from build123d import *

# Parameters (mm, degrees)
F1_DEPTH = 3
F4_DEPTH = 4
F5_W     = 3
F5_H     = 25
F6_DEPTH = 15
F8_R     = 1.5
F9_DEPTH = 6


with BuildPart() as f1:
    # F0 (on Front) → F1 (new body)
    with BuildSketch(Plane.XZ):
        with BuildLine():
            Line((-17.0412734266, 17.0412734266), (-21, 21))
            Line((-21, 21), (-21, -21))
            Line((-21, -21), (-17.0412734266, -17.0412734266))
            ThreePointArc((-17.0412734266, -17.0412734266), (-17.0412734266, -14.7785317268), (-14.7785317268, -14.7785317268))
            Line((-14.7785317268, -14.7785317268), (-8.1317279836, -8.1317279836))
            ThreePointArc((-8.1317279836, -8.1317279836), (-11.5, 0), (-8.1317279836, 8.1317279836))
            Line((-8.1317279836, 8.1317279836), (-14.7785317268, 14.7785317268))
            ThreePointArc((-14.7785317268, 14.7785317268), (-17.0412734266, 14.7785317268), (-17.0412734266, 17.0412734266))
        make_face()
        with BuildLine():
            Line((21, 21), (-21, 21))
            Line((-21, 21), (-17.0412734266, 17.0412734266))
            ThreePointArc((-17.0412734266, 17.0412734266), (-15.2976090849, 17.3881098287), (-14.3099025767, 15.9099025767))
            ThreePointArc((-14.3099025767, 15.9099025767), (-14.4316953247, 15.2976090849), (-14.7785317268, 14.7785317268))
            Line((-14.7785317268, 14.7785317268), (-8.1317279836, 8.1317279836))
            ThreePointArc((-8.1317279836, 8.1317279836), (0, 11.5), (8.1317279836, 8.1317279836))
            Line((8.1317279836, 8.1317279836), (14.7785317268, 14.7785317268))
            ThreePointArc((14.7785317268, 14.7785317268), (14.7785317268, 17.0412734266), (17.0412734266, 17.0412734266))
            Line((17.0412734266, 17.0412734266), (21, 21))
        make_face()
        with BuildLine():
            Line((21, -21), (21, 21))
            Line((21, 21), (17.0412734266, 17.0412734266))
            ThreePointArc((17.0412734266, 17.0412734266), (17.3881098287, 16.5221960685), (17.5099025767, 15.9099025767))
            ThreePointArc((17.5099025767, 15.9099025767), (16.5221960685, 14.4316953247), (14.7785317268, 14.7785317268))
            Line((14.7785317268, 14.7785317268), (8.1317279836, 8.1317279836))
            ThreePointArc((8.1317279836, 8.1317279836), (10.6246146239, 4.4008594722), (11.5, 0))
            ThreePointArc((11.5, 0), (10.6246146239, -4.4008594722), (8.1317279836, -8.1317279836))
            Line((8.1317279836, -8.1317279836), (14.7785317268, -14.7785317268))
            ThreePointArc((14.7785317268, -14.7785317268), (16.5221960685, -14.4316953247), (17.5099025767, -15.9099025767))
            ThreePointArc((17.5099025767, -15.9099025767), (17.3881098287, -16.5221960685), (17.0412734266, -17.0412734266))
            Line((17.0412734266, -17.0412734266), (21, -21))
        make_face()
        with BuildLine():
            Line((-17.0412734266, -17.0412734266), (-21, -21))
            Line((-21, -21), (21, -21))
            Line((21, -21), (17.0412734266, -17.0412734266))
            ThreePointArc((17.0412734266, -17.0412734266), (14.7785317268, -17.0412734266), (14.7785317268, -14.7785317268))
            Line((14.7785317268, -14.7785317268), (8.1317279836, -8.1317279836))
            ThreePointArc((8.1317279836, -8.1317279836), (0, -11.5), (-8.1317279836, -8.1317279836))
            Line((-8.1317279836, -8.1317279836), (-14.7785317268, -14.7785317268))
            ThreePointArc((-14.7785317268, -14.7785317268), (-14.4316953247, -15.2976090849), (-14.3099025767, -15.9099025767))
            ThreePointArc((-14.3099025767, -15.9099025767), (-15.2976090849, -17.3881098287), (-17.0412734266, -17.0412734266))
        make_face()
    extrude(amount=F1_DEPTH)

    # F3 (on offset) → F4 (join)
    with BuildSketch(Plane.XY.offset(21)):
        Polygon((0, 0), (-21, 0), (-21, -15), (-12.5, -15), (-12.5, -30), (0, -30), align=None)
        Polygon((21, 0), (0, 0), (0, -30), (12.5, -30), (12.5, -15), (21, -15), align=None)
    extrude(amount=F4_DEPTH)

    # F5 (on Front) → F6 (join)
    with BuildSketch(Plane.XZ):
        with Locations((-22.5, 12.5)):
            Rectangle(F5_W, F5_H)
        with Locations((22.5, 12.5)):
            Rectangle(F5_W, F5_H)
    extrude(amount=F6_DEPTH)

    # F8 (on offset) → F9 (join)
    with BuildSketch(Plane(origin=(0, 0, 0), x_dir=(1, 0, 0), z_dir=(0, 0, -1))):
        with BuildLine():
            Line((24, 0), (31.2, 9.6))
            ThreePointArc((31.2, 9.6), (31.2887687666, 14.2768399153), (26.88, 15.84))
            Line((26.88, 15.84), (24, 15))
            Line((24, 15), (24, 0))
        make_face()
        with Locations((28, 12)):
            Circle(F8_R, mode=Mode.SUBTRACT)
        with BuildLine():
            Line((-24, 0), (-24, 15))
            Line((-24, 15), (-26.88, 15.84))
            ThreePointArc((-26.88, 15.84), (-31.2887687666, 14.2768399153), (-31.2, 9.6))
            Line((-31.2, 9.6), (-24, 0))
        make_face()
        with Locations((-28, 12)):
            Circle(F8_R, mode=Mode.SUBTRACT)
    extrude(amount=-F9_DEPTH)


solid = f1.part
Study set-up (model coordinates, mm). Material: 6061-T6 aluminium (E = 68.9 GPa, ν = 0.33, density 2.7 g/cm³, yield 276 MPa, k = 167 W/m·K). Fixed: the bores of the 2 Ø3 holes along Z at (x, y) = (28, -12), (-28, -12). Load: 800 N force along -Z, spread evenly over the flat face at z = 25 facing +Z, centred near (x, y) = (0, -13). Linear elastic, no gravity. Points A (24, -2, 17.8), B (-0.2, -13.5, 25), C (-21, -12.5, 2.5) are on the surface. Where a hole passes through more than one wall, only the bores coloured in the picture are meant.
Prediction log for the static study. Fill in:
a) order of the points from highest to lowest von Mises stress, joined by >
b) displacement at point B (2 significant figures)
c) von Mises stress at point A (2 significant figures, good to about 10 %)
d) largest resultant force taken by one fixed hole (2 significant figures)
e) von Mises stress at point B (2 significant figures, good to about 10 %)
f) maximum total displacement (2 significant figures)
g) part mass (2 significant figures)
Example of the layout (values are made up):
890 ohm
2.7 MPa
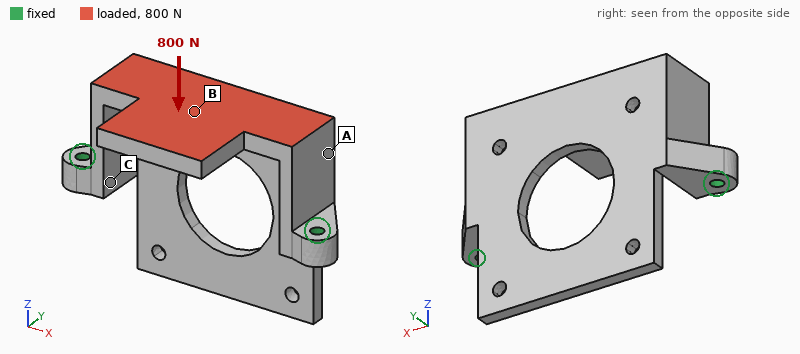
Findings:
B > A > C
0.062 mm
17 MPa
410 N
30 MPa
0.16 mm
30 g
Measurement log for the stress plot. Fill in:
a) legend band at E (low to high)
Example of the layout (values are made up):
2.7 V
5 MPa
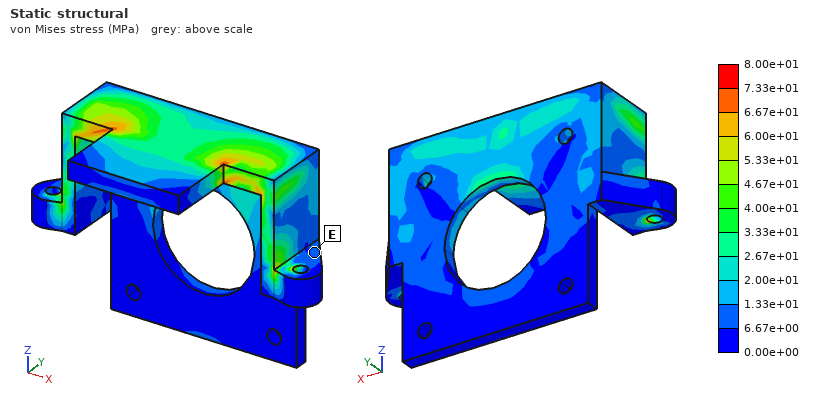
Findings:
6.67e+00 to 1.33e+01 MPa
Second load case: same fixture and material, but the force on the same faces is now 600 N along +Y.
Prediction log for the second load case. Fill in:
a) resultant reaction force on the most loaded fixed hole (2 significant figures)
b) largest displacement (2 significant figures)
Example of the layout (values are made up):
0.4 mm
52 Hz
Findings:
310 N
0.13 mm
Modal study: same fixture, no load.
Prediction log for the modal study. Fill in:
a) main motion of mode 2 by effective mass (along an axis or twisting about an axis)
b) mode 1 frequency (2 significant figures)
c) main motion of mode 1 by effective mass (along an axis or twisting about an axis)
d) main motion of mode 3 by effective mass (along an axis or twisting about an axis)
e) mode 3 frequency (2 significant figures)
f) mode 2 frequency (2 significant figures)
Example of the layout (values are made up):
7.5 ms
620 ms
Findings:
along Y
2400 Hz
twisting about X
along X
4500 Hz
3500 Hz
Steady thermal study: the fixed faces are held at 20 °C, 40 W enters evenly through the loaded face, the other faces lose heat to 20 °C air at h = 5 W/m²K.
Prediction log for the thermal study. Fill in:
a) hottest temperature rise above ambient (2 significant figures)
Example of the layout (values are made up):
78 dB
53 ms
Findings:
61 K
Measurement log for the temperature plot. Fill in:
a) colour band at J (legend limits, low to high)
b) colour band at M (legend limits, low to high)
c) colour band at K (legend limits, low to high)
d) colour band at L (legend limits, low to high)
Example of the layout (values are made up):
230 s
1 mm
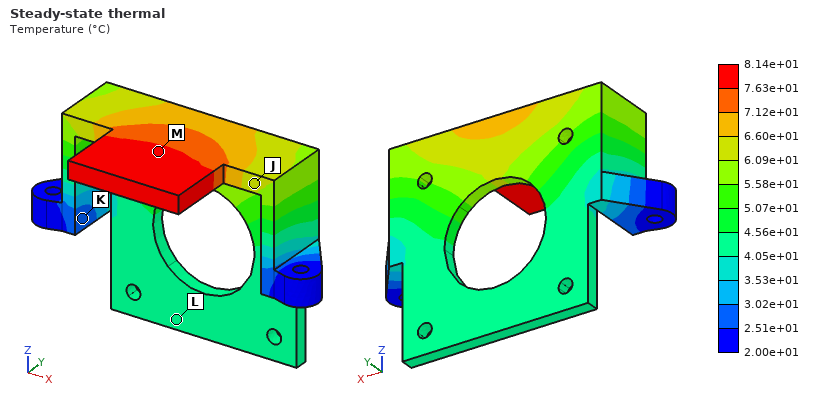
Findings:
6.09e+01 to 6.60e+01 °C
7.63e+01 to 8.14e+01 °C
2.51e+01 to 3.02e+01 °C
4.05e+01 to 4.56e+01 °C
